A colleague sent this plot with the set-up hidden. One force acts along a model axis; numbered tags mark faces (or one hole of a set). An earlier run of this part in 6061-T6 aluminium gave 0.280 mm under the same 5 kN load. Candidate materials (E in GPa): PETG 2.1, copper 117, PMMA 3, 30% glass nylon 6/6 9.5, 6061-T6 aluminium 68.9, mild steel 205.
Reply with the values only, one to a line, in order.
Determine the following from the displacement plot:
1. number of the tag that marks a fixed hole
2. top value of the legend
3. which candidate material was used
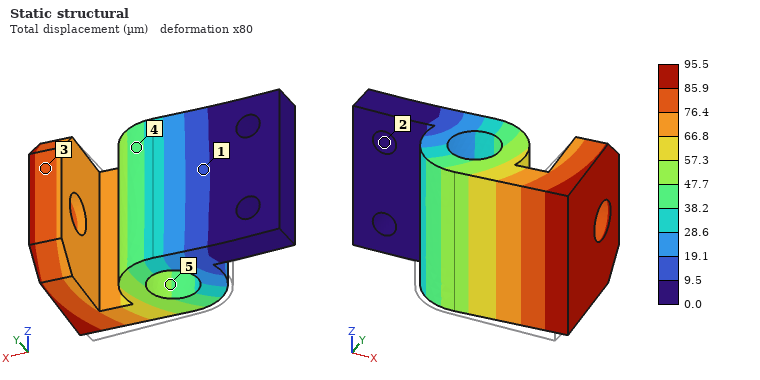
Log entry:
2
95.5 µm
mild steel
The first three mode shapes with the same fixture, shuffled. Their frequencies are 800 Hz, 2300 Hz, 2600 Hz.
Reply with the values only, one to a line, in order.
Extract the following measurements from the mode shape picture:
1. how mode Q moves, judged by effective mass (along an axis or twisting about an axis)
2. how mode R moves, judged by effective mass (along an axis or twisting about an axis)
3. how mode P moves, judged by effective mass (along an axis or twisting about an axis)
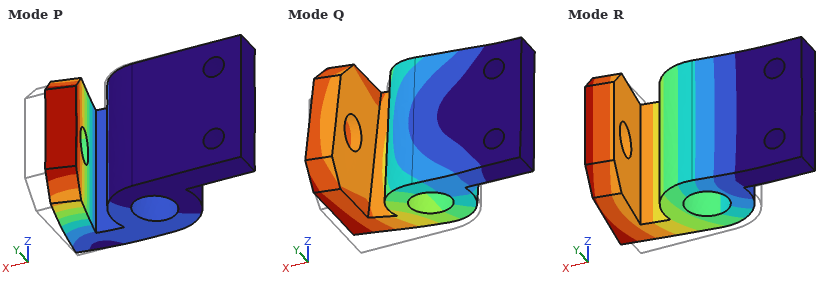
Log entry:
along Z
along Y
along X
